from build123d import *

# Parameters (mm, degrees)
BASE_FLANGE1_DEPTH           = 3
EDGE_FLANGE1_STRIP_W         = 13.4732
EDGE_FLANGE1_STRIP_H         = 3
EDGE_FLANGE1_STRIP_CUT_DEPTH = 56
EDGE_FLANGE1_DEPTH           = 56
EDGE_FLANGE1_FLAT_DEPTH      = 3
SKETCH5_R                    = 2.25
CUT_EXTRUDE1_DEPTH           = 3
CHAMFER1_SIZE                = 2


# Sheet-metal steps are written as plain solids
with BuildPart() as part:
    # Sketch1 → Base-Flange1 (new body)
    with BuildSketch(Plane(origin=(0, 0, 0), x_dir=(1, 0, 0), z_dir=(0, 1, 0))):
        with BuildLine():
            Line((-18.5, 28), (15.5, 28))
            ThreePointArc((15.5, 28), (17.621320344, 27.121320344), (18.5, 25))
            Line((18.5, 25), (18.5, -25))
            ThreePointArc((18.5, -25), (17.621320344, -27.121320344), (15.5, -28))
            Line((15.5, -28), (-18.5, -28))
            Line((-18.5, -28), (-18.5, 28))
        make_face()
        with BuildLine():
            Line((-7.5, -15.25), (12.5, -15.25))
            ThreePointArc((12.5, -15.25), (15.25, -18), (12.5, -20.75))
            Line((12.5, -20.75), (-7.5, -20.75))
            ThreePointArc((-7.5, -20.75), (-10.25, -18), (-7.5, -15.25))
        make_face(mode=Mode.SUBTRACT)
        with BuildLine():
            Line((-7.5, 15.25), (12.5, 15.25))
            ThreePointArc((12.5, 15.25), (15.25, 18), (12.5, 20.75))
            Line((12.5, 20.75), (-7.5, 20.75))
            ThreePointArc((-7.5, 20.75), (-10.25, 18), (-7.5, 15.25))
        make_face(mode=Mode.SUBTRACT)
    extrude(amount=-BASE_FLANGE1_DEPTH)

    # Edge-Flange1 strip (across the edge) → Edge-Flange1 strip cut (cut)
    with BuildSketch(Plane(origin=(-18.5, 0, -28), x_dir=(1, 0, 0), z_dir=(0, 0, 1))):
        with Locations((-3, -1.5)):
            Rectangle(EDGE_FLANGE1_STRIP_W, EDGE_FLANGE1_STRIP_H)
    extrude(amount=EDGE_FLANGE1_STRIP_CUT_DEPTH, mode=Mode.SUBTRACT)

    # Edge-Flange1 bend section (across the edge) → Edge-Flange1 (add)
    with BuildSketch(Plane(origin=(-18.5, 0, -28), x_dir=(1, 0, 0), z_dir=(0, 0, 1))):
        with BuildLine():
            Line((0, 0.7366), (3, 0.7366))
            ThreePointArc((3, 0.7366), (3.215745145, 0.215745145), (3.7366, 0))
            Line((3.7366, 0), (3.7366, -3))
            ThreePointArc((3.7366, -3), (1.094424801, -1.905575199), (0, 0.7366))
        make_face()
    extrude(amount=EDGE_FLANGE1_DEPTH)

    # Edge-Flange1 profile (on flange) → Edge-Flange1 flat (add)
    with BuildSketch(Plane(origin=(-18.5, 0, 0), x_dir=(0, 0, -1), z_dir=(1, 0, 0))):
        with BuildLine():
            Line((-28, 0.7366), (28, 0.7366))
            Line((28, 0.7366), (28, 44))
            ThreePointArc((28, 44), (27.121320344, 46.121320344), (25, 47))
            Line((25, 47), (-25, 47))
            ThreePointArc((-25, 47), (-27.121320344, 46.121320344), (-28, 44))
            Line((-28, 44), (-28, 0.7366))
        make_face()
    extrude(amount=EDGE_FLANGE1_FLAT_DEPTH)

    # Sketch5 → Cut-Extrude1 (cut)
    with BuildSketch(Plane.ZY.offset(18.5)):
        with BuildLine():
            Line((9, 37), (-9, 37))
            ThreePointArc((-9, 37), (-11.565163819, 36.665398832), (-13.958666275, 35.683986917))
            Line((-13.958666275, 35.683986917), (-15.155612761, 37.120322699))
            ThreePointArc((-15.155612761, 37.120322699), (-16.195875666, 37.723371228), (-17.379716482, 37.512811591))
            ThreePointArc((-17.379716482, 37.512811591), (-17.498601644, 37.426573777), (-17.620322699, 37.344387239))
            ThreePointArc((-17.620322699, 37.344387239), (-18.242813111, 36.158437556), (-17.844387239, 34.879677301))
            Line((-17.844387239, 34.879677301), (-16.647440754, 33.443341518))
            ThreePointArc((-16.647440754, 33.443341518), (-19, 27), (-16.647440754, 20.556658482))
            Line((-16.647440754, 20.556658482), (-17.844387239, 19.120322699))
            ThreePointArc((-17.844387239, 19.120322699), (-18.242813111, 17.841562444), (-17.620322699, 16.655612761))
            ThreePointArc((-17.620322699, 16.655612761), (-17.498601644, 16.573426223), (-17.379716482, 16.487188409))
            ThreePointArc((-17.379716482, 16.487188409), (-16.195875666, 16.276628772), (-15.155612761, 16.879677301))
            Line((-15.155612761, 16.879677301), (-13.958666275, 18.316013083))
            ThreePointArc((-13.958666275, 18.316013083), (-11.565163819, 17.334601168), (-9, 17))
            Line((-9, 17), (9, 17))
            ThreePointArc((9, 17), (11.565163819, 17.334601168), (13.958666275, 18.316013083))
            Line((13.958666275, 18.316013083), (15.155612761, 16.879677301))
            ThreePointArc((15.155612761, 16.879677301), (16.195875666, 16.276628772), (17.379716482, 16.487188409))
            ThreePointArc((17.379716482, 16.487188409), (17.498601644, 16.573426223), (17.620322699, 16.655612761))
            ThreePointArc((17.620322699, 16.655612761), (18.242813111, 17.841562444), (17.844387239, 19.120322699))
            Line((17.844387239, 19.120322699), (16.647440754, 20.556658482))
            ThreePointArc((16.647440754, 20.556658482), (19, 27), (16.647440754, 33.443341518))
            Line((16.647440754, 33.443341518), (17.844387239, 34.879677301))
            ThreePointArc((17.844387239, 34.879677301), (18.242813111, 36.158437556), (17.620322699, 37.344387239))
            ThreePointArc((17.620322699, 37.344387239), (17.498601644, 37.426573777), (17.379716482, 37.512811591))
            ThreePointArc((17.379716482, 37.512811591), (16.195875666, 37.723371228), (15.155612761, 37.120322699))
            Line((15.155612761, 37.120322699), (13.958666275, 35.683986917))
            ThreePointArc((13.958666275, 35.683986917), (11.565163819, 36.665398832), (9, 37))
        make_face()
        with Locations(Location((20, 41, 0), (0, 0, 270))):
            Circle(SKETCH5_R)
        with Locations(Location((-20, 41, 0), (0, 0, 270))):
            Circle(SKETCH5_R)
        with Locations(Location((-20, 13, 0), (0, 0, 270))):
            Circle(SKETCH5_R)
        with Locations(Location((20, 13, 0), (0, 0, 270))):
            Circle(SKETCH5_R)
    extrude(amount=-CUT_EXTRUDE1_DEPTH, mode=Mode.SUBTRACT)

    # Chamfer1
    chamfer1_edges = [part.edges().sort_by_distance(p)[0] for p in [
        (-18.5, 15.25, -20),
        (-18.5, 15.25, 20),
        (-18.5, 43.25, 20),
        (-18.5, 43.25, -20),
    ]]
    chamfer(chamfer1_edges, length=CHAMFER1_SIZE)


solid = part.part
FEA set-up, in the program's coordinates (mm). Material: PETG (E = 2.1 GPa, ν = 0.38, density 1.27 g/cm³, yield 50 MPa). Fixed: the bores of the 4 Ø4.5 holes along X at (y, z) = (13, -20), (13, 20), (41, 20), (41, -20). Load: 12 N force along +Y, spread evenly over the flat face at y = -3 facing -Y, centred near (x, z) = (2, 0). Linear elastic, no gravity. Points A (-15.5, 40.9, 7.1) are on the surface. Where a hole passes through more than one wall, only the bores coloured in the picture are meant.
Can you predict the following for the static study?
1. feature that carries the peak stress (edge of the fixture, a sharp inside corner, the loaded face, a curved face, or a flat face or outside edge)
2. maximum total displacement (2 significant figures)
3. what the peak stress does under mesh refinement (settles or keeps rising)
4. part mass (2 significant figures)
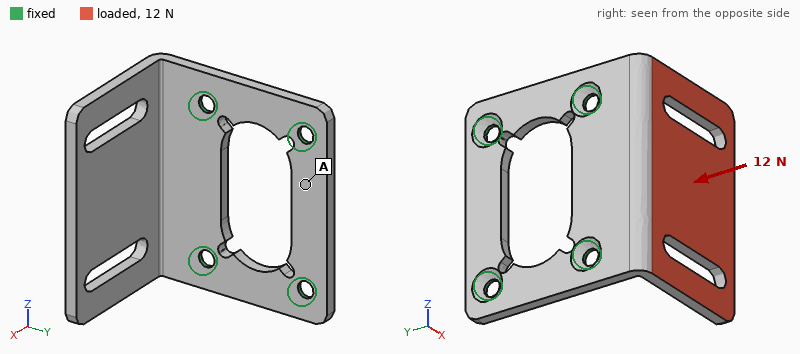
edge of the fixture
0.94 mm
keeps rising
14 g
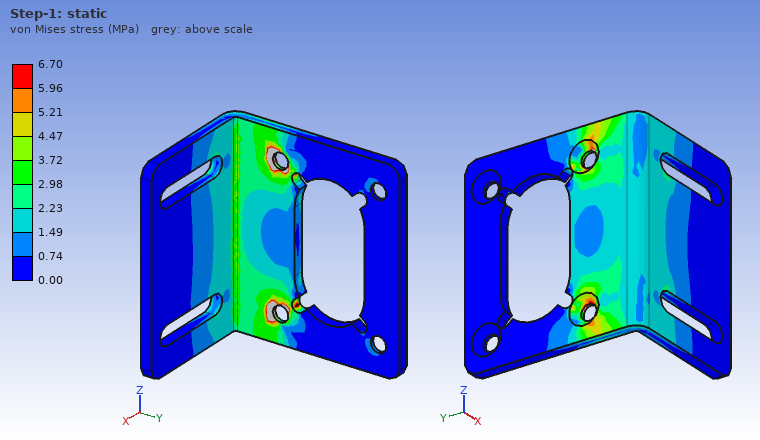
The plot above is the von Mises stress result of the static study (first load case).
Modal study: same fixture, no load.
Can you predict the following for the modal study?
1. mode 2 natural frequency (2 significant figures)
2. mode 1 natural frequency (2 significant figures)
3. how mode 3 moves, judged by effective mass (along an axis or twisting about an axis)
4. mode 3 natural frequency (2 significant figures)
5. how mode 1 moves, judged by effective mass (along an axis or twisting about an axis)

610 Hz
270 Hz
along X
930 Hz
along Y
